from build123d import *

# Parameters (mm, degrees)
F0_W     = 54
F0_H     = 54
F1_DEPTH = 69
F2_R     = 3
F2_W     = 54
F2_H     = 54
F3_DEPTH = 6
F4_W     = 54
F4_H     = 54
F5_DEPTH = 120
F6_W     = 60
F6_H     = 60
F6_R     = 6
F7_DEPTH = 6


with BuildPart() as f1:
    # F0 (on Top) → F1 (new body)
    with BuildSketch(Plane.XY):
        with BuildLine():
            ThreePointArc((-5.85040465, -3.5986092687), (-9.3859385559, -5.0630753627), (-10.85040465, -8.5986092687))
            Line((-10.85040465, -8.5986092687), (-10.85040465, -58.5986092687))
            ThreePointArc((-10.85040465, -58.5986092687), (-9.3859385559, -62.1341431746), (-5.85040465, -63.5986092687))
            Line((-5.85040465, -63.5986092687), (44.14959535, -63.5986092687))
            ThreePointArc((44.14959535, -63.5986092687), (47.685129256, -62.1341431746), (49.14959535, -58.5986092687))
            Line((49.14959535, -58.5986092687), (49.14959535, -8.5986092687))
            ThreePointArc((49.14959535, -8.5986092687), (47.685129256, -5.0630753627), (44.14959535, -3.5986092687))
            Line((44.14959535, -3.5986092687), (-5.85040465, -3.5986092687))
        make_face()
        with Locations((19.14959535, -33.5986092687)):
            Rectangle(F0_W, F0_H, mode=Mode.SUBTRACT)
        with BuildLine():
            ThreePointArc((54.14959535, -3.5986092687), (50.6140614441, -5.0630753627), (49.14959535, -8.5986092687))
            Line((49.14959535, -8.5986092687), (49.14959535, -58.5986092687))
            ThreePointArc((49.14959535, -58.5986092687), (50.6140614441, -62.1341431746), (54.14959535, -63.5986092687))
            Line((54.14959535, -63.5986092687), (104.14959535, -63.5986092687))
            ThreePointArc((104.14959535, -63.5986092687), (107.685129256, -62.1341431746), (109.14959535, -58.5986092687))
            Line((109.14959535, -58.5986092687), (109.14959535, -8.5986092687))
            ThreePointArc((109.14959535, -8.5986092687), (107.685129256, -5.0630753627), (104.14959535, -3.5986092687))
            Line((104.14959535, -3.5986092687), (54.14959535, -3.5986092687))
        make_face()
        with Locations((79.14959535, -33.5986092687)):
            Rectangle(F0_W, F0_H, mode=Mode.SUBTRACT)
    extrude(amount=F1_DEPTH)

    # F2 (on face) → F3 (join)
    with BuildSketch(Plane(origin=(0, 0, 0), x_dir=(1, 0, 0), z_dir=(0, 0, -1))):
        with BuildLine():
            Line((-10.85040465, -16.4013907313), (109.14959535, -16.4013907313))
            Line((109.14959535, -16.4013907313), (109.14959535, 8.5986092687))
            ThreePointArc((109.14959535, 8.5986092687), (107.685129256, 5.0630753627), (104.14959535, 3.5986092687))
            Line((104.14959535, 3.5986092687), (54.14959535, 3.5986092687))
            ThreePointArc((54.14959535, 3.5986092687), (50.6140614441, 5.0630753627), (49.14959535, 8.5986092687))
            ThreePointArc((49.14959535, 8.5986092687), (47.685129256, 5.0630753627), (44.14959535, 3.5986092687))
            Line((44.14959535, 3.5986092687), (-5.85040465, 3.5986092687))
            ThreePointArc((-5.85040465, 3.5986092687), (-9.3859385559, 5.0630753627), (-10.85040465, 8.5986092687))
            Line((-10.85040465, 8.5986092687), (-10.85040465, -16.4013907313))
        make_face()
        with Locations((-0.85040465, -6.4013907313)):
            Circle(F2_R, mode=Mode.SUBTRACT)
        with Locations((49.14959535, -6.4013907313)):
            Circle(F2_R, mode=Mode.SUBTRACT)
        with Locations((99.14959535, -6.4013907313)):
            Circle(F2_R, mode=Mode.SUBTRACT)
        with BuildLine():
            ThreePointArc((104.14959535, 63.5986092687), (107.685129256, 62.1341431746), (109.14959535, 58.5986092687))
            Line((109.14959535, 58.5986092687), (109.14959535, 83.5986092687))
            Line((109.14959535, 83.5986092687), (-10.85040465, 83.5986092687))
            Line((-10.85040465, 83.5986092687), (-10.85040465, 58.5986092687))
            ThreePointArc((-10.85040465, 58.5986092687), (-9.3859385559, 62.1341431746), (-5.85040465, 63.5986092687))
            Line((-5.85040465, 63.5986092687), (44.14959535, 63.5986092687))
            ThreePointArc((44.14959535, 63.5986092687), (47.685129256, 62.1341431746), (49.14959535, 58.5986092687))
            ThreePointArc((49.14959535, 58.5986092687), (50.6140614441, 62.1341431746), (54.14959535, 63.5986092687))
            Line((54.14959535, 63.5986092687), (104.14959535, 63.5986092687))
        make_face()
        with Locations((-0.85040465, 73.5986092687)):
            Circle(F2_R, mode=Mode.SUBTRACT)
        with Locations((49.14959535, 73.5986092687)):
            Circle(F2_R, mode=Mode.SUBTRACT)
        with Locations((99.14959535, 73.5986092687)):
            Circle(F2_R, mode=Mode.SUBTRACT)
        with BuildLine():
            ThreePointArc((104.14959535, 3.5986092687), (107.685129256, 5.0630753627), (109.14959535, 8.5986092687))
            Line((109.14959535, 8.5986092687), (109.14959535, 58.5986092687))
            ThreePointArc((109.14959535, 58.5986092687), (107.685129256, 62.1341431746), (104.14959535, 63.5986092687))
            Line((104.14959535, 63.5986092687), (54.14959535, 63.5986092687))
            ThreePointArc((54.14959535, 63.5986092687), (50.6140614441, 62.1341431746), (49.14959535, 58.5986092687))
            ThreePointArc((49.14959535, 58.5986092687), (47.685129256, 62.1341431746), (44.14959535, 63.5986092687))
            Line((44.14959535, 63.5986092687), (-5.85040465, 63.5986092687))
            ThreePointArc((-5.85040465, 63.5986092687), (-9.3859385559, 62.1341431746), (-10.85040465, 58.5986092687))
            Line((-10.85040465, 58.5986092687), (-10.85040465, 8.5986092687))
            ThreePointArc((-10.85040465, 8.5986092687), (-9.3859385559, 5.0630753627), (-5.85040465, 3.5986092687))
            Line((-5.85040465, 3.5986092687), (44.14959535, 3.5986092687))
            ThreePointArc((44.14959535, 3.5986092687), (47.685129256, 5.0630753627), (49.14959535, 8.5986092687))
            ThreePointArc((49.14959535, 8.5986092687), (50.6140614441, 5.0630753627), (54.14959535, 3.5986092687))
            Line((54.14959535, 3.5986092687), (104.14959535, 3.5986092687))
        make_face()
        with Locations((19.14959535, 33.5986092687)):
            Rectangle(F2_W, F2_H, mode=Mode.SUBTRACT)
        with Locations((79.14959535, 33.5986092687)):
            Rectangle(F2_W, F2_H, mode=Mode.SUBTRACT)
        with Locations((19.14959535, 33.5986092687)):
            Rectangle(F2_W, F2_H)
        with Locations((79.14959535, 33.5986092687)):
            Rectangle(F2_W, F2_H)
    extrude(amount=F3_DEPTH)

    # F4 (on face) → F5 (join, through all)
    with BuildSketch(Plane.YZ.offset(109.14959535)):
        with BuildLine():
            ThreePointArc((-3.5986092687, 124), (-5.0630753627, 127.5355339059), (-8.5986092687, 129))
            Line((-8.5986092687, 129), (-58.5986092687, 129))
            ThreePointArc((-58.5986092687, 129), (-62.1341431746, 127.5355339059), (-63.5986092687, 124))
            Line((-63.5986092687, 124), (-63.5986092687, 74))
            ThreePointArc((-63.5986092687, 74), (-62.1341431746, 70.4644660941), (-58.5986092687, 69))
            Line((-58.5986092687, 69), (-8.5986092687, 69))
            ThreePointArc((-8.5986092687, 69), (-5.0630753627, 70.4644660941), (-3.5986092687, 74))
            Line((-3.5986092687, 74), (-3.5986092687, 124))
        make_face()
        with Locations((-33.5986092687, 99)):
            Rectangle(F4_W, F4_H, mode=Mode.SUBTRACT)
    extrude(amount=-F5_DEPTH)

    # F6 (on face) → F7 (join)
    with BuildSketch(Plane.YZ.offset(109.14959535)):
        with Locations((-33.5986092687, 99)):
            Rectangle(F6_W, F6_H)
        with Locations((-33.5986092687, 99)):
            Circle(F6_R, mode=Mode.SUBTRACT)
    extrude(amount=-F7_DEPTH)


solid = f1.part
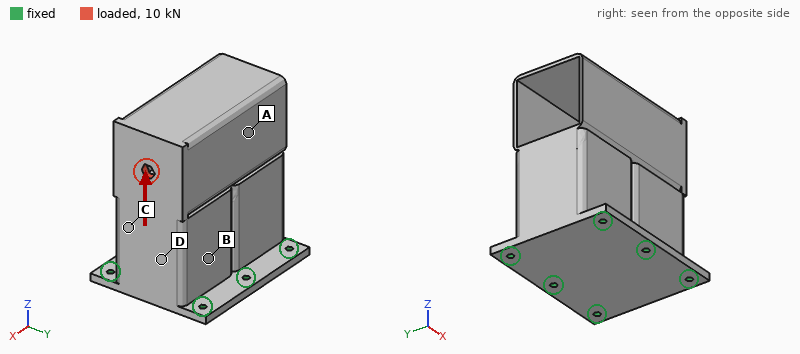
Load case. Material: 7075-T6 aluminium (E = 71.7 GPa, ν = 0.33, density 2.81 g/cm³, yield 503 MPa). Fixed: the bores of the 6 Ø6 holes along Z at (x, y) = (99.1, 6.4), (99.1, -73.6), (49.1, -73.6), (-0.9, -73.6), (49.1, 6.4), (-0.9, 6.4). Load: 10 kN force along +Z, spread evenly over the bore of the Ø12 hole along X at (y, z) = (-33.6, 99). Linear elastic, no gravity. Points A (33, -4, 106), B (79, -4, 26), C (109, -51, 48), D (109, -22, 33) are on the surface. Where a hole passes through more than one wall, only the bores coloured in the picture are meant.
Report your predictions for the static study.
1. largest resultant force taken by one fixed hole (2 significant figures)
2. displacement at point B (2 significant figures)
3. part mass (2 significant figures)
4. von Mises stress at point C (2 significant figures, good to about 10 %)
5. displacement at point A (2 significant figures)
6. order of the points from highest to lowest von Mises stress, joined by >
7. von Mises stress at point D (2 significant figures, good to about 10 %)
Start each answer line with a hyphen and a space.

- 4.7 kN
- 0.049 mm
- 730 g
- 40 MPa
- 0.11 mm
- C > D > B > A
- 32 MPa
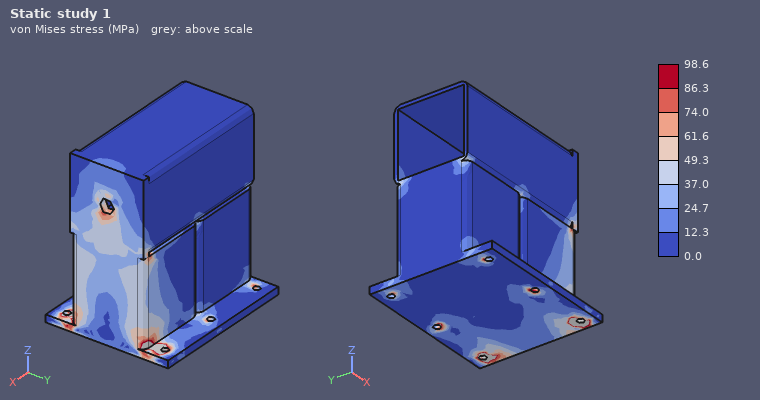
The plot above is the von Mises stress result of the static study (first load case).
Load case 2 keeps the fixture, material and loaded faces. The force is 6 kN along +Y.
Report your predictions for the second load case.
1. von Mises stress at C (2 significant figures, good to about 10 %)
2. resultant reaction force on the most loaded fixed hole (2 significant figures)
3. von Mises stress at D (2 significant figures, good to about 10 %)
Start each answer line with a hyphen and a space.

- 39 MPa
- 4.3 kN
- 36 MPa
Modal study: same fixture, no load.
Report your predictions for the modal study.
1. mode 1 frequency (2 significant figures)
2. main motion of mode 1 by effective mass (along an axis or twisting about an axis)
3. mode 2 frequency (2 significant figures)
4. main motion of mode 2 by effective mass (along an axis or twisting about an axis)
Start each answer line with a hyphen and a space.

- 1200 Hz
- along Y
- 1600 Hz
- along X
